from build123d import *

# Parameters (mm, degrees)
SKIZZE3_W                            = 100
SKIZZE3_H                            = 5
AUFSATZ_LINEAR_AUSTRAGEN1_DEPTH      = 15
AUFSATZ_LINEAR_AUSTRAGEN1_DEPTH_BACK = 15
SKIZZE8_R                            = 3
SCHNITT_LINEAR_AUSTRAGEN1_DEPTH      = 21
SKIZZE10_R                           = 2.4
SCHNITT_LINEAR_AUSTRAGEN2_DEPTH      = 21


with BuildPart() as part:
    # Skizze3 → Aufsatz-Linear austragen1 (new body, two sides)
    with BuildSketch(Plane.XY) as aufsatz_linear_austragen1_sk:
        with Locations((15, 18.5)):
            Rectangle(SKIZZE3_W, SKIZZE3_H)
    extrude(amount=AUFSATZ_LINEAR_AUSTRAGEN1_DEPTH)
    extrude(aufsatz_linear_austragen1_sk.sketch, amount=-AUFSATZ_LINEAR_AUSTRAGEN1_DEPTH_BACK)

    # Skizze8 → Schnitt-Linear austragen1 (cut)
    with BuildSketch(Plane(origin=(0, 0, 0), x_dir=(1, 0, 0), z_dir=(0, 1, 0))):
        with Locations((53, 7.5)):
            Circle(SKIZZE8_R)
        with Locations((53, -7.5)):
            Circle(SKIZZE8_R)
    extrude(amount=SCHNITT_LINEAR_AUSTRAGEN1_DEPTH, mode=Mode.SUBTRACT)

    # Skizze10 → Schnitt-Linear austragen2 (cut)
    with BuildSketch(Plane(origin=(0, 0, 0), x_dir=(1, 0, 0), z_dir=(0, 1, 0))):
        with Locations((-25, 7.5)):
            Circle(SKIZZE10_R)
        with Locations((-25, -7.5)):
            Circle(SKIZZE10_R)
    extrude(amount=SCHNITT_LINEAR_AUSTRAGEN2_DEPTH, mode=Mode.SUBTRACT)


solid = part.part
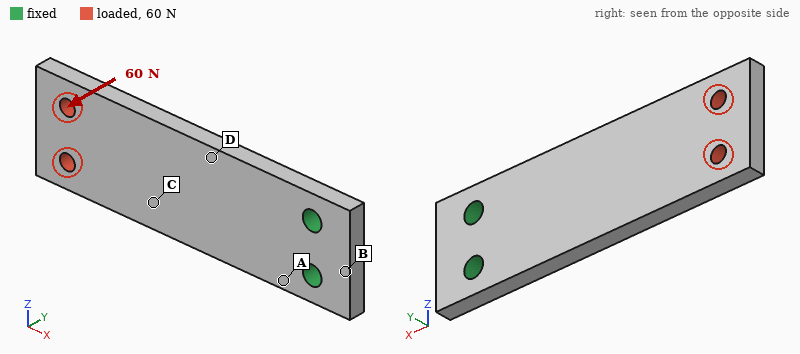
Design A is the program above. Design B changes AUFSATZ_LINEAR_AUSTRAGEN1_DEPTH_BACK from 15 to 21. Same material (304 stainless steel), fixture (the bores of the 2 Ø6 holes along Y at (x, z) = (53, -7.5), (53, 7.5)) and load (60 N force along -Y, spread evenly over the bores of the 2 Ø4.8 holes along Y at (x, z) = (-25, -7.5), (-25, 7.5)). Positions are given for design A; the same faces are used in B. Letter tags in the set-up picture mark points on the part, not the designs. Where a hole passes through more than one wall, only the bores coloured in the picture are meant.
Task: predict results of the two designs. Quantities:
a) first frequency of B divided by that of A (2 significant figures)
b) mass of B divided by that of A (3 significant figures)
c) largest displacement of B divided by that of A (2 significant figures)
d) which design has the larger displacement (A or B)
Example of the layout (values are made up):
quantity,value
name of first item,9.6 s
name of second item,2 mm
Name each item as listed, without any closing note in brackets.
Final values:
quantity,value
first frequency of B divided by that of A,0.99
mass of B divided by that of A,1.21
largest displacement of B divided by that of A,0.85
which design has the larger displacement,A
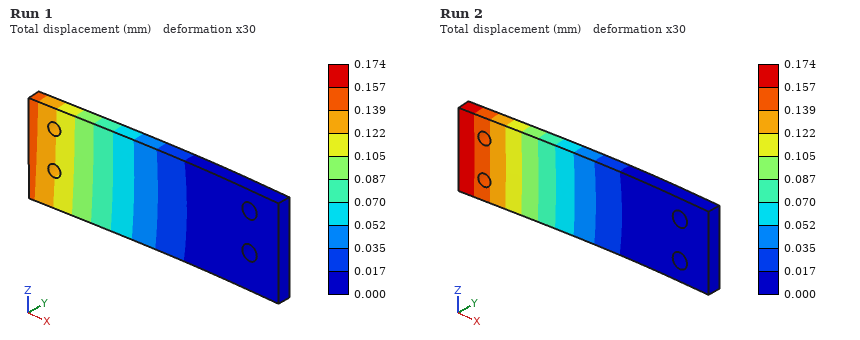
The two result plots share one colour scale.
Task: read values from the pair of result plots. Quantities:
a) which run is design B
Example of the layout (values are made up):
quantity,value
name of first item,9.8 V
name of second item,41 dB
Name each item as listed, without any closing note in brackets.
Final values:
quantity,value
which run is design B,Run 1
